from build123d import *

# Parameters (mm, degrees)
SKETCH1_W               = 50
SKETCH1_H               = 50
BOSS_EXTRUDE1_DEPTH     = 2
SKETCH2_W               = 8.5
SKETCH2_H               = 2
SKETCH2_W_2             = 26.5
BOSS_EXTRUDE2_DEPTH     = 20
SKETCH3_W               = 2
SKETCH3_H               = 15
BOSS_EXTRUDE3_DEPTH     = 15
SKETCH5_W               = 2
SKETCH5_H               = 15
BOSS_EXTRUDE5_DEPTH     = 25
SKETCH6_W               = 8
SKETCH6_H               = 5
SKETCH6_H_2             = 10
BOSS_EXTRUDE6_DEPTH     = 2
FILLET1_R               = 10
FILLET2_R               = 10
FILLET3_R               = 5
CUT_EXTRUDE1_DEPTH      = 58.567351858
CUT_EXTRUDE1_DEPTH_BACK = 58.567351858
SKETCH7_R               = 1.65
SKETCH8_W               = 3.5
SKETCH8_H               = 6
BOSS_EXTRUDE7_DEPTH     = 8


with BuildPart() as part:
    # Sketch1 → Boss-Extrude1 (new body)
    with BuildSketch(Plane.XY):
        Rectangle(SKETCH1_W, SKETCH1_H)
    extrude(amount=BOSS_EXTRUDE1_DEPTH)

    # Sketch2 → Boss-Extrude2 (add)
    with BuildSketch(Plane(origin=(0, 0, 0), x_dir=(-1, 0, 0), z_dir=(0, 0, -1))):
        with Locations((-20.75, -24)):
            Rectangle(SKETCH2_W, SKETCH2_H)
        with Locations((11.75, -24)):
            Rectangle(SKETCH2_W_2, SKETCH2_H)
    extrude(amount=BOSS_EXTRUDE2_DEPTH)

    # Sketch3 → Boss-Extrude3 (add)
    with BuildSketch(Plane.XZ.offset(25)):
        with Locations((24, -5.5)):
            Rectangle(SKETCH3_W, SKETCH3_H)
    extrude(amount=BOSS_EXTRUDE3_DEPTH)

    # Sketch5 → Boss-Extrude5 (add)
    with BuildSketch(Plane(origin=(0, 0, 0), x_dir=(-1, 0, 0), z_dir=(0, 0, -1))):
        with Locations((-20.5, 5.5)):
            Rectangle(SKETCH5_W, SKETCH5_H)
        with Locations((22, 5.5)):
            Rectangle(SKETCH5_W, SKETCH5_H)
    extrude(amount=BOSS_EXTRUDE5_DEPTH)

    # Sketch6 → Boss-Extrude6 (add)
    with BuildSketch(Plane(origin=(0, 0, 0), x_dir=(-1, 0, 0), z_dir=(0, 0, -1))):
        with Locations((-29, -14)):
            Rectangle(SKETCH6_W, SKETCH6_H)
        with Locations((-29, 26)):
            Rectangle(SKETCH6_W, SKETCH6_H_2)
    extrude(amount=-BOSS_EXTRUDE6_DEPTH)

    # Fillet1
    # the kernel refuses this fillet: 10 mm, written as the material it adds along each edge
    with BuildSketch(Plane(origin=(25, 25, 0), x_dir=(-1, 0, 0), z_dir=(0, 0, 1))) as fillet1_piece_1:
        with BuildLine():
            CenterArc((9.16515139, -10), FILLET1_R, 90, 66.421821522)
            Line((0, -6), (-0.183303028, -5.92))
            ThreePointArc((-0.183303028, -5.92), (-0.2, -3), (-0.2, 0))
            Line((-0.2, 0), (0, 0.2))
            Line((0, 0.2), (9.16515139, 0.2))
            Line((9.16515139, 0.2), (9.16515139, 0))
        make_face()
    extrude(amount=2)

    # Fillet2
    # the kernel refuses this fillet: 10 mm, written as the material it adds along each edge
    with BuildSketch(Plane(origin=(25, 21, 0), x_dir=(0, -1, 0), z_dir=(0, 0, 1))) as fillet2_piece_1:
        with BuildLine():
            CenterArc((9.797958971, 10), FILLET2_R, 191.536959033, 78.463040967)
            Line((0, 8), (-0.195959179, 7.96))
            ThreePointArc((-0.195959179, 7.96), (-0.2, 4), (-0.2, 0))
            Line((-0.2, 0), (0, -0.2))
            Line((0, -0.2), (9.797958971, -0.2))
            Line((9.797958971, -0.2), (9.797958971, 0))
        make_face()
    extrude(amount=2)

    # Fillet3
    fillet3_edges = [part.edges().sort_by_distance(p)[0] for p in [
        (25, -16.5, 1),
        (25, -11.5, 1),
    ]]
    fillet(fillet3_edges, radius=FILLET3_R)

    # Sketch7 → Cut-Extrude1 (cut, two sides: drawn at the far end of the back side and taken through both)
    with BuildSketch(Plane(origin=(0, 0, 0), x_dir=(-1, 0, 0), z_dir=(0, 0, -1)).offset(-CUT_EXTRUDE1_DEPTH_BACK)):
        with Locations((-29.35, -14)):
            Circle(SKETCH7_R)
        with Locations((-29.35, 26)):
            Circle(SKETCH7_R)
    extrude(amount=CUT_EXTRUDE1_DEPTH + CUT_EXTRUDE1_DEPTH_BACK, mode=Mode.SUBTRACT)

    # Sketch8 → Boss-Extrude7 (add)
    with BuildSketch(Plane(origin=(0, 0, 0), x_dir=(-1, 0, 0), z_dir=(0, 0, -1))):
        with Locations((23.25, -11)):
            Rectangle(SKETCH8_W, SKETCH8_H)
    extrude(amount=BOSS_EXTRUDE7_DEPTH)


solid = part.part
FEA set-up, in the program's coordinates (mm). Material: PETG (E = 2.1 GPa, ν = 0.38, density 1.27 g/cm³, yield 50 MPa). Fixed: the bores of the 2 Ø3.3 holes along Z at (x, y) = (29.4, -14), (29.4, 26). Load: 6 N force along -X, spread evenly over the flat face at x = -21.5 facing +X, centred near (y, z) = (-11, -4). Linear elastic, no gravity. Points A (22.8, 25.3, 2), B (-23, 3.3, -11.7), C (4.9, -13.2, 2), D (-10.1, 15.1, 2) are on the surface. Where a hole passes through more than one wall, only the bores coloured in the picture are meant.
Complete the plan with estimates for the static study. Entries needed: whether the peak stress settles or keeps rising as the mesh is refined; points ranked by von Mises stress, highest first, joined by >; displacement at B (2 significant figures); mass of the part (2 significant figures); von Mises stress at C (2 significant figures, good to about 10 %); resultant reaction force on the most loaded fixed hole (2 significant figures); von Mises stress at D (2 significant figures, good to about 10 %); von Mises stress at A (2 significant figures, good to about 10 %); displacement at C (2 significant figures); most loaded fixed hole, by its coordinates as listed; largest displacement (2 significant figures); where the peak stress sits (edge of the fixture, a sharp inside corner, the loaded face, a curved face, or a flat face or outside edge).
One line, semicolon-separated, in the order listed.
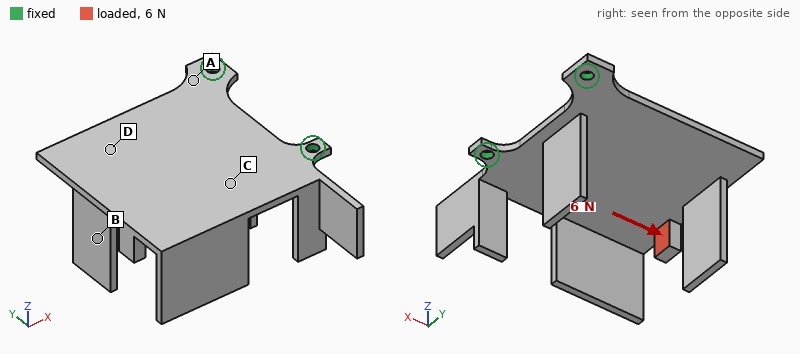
keeps rising; A > C > D > B; 0.85 mm; 11 g; 0.88 MPa; 5.5 N; 0.55 MPa; 1.7 MPa; 0.25 mm; (29.4, -14); 1.0 mm; edge of the fixture
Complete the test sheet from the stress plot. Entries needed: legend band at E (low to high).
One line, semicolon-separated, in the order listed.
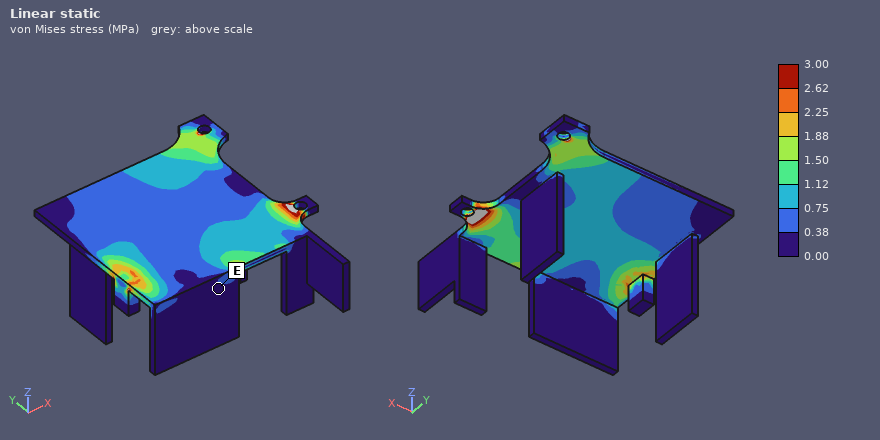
0.00 to 0.38 MPa
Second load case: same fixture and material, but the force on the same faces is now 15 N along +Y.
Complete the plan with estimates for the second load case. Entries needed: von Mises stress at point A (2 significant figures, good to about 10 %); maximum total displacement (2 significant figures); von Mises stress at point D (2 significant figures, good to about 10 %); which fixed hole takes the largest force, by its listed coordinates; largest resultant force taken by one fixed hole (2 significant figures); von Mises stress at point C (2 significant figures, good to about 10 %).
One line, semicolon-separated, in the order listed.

3.1 MPa; 1.1 mm; 0.99 MPa; (29.4, 26); 22 N; 1.7 MPa
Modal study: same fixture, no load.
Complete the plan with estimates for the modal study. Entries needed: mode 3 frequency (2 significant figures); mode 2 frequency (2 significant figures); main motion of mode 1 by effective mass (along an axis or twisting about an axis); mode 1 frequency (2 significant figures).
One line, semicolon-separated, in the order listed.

390 Hz; 210 Hz; along Z; 75 Hz
